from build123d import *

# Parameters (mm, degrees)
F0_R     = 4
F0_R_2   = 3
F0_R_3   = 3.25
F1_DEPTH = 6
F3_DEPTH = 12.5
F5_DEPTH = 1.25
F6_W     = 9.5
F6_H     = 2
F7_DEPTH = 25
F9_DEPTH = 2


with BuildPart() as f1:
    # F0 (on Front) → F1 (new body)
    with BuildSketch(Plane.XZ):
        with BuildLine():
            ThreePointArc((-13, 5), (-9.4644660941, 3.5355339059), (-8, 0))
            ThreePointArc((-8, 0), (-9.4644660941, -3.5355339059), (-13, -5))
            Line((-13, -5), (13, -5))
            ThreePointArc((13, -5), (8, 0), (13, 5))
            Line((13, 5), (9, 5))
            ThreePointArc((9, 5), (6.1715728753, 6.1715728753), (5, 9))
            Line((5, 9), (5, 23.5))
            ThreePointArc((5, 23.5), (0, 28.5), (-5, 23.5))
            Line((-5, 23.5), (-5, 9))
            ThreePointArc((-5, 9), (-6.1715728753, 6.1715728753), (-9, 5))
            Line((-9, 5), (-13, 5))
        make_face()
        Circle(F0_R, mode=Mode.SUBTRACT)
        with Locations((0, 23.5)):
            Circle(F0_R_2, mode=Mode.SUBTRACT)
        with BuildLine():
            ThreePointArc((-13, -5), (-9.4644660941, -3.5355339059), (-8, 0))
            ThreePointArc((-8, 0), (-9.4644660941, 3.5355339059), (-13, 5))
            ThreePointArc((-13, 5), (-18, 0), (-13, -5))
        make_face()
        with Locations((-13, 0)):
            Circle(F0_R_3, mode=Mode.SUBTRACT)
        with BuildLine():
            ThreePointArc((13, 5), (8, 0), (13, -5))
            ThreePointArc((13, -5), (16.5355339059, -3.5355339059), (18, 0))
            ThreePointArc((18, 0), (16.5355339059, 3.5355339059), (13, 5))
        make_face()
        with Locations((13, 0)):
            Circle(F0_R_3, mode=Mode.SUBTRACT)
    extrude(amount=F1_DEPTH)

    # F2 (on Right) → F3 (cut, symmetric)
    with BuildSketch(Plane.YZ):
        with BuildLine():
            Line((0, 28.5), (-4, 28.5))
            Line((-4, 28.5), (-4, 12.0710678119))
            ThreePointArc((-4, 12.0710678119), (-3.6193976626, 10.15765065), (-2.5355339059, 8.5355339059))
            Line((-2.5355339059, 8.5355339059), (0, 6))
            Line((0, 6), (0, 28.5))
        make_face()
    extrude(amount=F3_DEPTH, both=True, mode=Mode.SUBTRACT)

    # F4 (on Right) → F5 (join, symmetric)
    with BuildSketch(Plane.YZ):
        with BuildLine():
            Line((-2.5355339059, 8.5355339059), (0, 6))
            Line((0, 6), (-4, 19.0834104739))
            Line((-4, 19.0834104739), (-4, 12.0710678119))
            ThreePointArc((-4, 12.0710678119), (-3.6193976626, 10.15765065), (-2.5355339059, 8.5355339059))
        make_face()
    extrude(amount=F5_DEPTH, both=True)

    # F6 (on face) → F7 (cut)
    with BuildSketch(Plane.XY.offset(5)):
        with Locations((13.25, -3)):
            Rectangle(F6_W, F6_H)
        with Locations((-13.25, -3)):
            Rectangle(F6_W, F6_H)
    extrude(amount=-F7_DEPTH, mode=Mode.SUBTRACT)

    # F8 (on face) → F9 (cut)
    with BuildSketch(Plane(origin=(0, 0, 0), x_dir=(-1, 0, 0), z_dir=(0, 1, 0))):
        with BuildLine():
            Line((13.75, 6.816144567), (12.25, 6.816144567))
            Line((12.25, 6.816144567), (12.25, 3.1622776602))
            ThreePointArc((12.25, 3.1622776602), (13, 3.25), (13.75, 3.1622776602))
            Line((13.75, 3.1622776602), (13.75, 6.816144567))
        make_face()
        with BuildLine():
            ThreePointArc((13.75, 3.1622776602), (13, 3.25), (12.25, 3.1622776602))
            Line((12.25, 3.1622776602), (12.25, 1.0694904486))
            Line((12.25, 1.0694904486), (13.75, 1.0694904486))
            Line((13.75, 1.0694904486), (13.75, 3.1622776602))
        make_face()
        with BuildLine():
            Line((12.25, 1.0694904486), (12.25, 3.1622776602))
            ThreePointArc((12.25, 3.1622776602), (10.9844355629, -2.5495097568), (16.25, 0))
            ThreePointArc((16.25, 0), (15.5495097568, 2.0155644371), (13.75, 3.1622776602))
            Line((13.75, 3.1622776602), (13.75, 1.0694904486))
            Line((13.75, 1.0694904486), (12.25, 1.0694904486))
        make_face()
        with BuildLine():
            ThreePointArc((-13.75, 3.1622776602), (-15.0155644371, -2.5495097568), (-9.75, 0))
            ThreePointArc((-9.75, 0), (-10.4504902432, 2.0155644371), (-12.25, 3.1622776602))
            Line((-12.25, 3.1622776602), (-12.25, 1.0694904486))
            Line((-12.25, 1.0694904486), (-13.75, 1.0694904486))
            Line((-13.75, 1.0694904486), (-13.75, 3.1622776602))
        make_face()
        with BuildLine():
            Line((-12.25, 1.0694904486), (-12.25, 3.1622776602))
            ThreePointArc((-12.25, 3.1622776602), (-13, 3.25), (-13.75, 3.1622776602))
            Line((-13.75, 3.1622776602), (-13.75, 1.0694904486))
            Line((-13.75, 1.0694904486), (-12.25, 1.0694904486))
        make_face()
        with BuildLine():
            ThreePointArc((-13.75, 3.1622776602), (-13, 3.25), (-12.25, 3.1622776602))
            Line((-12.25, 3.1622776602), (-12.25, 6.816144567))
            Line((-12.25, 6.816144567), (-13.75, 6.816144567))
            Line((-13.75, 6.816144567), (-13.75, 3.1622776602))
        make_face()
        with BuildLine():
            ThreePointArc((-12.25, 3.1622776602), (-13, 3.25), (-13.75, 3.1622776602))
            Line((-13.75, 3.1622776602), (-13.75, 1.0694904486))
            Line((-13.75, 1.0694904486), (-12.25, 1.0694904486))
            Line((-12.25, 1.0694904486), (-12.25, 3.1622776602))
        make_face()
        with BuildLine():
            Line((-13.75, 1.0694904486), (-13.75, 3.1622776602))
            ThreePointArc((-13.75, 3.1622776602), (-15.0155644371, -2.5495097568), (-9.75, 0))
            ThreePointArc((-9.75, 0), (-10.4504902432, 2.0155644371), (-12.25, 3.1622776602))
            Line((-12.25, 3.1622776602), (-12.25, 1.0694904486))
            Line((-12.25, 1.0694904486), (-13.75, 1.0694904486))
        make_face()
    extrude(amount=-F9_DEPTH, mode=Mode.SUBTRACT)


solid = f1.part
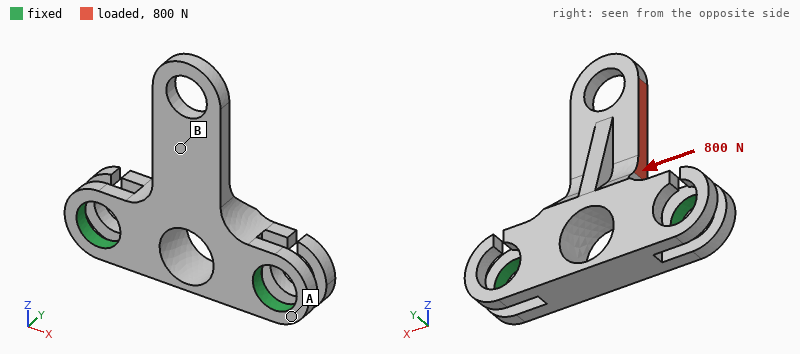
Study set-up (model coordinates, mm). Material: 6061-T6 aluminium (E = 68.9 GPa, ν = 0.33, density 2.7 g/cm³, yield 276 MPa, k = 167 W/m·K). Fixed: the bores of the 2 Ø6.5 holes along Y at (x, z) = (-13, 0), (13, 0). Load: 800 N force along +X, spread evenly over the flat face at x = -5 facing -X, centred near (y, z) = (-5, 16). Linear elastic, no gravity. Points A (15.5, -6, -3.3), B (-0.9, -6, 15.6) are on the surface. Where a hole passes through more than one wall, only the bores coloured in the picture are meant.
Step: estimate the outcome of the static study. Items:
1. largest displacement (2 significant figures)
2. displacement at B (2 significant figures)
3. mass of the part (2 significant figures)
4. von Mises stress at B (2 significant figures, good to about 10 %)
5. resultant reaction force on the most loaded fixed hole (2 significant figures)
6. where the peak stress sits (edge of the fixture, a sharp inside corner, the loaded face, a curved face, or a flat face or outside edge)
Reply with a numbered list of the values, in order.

1. 0.11 mm
2. 0.044 mm
3. 4.6 g
4. 56 MPa
5. 770 N
6. a curved face
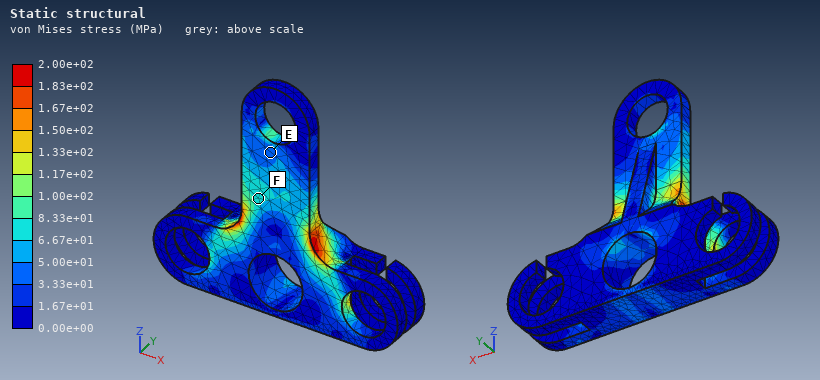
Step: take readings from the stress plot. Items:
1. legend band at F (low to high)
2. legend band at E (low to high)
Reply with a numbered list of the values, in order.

1. 6.67e+01 to 8.33e+01 MPa
2. 3.33e+01 to 5.00e+01 MPa
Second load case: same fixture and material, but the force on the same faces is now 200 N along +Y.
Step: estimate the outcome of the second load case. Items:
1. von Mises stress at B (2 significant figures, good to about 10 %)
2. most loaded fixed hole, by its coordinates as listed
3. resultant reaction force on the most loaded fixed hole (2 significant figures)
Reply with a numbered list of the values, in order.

1. 76 MPa
2. (-13, 0)
3. 200 N
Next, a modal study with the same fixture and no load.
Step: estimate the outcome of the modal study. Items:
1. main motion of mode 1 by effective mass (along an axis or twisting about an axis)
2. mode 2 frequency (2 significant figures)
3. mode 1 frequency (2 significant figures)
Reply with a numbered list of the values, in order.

1. along Y
2. 7200 Hz
3. 5700 Hz
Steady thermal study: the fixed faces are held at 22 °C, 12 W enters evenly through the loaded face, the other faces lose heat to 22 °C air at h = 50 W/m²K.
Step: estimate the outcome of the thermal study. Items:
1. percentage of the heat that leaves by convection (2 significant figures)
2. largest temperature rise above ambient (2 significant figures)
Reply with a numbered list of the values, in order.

1. 8.8 %
2. 46 K
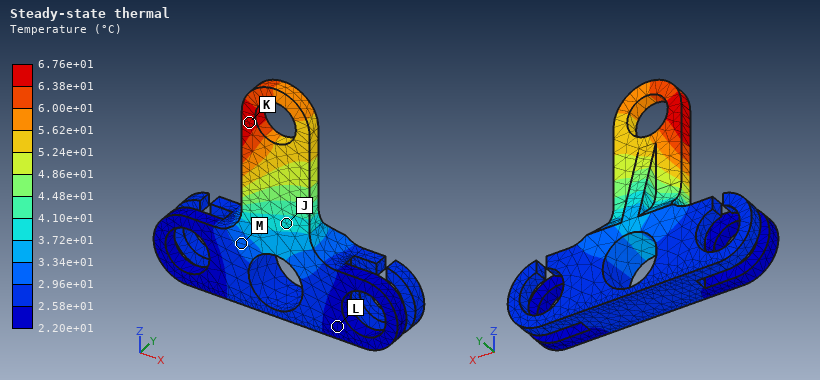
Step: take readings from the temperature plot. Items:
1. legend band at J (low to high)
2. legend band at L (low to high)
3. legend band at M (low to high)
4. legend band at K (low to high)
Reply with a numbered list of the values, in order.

1. 3.72e+01 to 4.10e+01 °C
2. 2.20e+01 to 2.58e+01 °C
3. 2.96e+01 to 3.34e+01 °C
4. 6.38e+01 to 6.76e+01 °C
